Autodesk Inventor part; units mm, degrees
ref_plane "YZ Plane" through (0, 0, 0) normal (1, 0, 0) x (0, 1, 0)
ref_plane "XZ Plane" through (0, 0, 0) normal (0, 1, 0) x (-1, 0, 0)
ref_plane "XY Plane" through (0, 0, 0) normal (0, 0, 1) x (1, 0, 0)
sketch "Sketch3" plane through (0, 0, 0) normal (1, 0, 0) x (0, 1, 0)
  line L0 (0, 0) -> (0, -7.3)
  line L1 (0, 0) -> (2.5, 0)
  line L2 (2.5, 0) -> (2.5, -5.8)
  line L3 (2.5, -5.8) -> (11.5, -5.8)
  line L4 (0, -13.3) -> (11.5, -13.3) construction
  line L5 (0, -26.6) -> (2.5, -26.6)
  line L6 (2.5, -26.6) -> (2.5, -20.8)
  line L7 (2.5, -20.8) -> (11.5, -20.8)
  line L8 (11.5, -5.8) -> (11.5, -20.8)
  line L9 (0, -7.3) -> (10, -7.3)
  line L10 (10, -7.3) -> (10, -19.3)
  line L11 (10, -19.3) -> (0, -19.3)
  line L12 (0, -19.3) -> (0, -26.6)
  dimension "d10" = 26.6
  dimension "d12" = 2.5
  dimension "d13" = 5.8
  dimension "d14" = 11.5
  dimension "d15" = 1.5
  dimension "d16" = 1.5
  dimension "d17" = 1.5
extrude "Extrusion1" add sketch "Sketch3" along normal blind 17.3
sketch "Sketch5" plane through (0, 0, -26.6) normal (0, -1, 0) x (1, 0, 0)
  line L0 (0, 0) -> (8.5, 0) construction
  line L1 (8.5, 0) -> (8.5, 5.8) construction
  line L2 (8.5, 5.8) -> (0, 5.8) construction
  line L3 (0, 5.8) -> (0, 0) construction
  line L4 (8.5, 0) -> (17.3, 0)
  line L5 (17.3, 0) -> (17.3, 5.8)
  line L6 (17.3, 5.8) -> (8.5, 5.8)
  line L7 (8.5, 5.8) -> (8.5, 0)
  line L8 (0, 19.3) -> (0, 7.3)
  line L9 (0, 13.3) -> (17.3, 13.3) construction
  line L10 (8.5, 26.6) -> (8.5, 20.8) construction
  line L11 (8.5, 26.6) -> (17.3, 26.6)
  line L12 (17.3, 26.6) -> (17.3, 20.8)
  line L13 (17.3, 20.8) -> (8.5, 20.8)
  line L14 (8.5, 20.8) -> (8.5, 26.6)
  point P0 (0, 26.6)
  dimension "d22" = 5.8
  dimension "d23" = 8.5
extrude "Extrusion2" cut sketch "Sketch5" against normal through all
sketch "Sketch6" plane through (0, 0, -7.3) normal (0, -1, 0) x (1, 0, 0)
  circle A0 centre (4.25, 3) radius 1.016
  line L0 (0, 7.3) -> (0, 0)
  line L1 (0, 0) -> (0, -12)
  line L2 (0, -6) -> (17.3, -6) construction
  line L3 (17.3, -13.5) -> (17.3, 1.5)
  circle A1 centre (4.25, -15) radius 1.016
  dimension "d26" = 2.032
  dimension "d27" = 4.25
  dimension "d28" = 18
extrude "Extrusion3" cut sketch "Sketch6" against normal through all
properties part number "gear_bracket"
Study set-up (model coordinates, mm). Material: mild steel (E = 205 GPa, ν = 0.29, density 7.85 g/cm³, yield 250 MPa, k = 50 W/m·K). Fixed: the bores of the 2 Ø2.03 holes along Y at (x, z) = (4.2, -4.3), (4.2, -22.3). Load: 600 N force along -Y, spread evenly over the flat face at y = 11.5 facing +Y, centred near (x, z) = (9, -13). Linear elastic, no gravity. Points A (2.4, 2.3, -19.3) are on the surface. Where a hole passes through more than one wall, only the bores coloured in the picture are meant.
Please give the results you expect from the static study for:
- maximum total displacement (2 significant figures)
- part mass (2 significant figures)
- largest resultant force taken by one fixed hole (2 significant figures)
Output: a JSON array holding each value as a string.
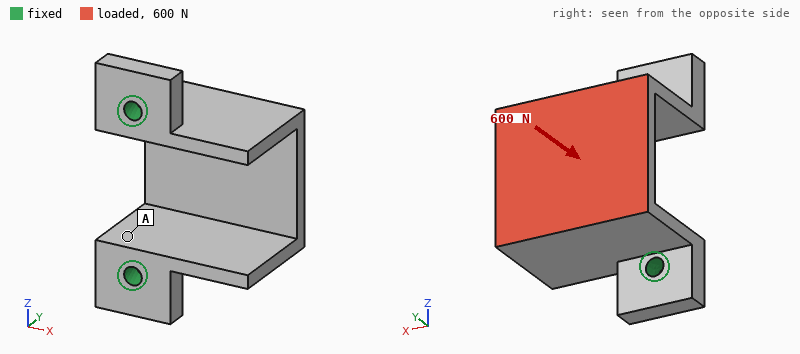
["26 µm", "8.9 g", "310 N"]
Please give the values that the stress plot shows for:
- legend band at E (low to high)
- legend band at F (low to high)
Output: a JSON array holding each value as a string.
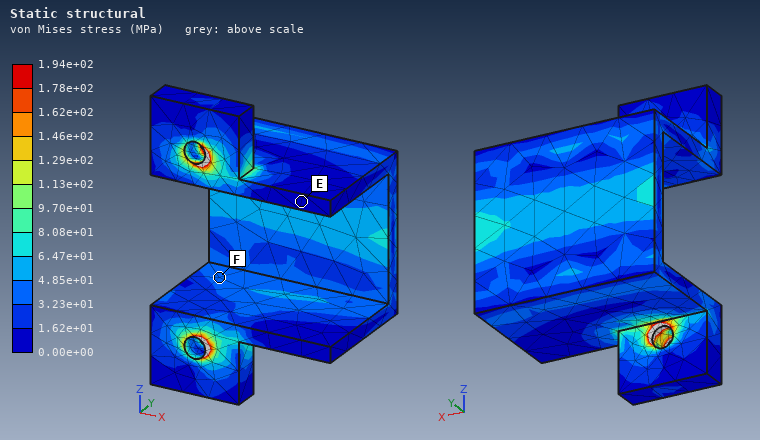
["0.00e+00 to 1.62e+01 MPa", "3.23e+01 to 4.85e+01 MPa"]
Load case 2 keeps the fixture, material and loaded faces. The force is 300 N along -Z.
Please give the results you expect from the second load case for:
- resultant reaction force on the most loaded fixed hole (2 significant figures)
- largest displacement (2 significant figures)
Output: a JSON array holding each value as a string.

["200 N", "23 µm"]
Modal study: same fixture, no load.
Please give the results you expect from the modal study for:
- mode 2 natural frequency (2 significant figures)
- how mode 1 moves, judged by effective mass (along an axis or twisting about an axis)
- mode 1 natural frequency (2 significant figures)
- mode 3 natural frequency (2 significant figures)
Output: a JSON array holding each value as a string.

["9400 Hz", "along Z", "8700 Hz", "12 kHz"]
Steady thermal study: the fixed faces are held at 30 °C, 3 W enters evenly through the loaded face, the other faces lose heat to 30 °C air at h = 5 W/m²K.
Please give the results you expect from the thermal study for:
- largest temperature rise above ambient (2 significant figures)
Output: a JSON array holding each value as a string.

["20 K"]
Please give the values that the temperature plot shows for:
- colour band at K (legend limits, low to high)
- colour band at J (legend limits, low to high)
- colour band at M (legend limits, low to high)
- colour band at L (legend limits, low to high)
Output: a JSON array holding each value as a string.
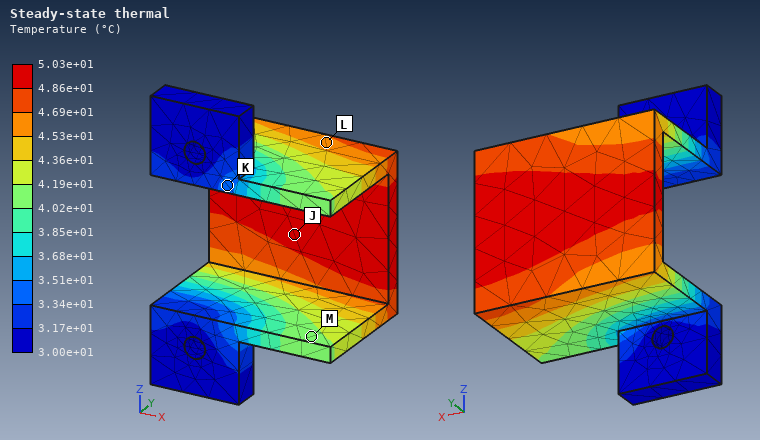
["3.34e+01 to 3.51e+01 °C", "4.86e+01 to 5.03e+01 °C", "4.02e+01 to 4.19e+01 °C", "4.53e+01 to 4.69e+01 °C"]
